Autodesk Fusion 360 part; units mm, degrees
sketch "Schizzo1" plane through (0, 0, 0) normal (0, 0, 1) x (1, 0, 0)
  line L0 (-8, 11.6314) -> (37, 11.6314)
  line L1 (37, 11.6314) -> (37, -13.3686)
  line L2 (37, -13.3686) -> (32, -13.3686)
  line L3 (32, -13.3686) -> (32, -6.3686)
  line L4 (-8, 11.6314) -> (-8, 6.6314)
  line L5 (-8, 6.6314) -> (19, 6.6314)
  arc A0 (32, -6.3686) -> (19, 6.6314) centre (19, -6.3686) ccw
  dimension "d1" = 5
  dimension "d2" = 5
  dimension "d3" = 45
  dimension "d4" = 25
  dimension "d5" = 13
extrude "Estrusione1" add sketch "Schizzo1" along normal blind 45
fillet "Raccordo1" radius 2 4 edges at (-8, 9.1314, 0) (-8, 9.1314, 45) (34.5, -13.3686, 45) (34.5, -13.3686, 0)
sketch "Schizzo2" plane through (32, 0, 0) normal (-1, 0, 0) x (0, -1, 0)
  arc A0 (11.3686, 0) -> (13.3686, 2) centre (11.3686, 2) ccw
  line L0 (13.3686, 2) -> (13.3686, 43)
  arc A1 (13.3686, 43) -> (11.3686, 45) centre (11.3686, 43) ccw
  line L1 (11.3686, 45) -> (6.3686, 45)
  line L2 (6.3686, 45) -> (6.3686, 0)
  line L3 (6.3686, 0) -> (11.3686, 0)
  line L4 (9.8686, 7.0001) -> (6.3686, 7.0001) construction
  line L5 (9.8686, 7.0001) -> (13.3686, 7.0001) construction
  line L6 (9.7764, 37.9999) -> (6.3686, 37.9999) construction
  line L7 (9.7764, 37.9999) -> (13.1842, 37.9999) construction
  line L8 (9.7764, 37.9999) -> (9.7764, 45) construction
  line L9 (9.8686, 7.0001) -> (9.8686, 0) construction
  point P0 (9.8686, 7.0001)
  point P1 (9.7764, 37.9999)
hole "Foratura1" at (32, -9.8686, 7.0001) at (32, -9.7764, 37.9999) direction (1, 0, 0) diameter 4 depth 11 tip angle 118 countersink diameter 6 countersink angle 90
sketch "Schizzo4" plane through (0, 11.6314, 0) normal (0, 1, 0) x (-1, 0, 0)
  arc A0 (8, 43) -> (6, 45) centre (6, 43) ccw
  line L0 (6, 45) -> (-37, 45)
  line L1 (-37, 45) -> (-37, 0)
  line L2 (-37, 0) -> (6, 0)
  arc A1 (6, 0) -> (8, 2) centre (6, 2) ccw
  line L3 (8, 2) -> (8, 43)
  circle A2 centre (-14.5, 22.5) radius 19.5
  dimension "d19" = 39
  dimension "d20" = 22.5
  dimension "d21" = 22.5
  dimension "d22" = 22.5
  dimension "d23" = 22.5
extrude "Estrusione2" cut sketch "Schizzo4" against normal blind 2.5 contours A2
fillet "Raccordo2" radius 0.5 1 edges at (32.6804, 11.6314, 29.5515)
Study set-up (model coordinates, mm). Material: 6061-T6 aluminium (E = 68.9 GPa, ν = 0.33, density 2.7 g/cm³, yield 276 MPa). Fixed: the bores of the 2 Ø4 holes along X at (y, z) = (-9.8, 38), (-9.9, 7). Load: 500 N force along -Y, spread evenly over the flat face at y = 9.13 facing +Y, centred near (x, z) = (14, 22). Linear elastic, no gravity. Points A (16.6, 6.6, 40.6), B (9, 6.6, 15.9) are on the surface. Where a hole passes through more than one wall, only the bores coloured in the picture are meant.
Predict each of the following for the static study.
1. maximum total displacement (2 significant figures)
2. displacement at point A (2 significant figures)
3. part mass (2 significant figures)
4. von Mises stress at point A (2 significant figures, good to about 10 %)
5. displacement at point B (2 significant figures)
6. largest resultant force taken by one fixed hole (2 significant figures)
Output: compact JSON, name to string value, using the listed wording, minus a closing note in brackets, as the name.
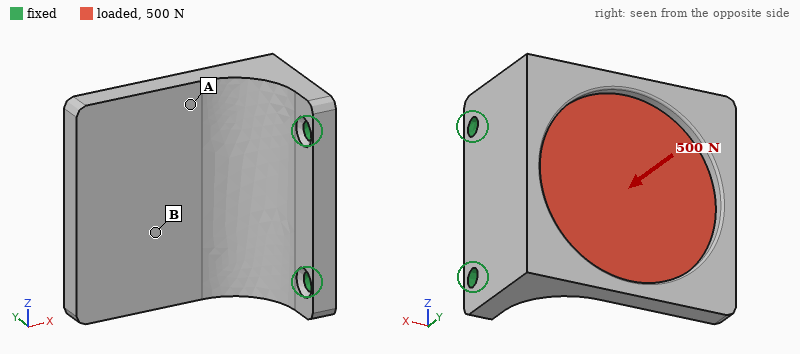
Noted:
{"maximum total displacement": "0.32 mm", "displacement at point A": "0.100 mm", "part mass": "35 g", "von Mises stress at point A": "29 MPa", "displacement at point B": "0.16 mm", "largest resultant force taken by one fixed hole": "270 N"}
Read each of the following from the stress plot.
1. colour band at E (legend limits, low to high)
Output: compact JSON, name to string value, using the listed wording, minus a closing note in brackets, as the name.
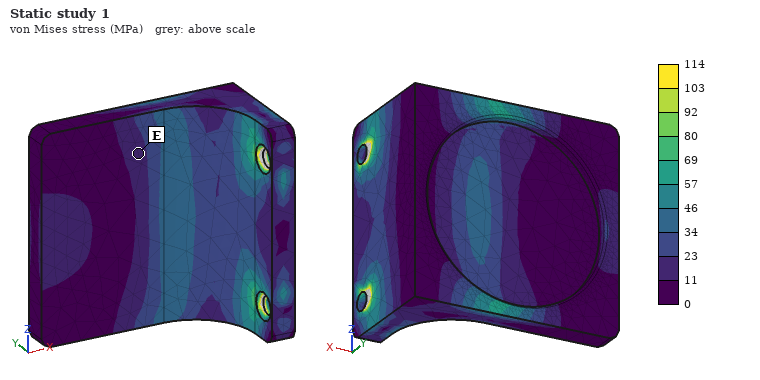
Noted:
{"colour band at E": "11 to 23 MPa"}
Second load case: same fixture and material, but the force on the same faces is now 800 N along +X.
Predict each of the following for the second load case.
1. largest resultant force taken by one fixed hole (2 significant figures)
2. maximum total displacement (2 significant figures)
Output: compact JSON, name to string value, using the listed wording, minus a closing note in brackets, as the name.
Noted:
{"largest resultant force taken by one fixed hole": "400 N", "maximum total displacement": "0.24 mm"}
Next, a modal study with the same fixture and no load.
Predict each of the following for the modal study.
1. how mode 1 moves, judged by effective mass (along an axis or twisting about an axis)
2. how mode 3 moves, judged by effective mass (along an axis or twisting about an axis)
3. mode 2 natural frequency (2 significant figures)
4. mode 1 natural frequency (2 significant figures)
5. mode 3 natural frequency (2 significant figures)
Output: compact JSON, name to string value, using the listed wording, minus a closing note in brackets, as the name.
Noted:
{"how mode 1 moves, judged by effective mass": "along Y", "how mode 3 moves, judged by effective mass": "along X", "mode 2 natural frequency": "3700 Hz", "mode 1 natural frequency": "1600 Hz", "mode 3 natural frequency": "4600 Hz"}
